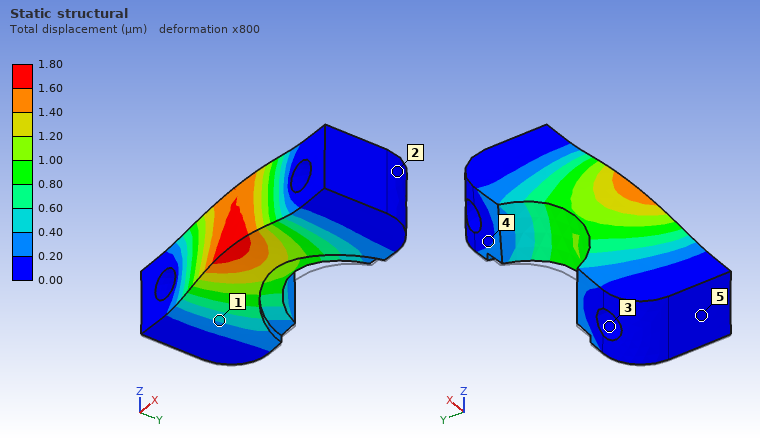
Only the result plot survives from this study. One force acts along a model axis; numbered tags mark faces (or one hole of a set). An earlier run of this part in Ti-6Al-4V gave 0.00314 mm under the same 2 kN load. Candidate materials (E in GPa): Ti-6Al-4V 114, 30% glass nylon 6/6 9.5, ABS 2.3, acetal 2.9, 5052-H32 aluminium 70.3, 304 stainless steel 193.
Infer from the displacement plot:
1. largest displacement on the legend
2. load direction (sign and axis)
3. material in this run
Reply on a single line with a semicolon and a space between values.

1.80 µm; +Z; 304 stainless steel
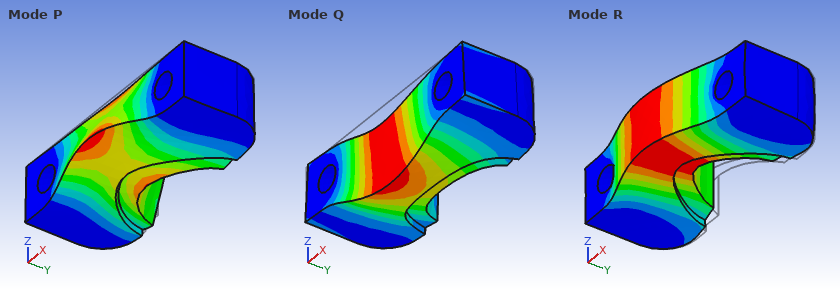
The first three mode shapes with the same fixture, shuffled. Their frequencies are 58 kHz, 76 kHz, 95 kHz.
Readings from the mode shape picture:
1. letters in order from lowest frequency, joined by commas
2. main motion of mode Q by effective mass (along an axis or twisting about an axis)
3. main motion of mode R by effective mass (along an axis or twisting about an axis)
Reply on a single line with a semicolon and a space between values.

Q, R, P; along Z; along Y
